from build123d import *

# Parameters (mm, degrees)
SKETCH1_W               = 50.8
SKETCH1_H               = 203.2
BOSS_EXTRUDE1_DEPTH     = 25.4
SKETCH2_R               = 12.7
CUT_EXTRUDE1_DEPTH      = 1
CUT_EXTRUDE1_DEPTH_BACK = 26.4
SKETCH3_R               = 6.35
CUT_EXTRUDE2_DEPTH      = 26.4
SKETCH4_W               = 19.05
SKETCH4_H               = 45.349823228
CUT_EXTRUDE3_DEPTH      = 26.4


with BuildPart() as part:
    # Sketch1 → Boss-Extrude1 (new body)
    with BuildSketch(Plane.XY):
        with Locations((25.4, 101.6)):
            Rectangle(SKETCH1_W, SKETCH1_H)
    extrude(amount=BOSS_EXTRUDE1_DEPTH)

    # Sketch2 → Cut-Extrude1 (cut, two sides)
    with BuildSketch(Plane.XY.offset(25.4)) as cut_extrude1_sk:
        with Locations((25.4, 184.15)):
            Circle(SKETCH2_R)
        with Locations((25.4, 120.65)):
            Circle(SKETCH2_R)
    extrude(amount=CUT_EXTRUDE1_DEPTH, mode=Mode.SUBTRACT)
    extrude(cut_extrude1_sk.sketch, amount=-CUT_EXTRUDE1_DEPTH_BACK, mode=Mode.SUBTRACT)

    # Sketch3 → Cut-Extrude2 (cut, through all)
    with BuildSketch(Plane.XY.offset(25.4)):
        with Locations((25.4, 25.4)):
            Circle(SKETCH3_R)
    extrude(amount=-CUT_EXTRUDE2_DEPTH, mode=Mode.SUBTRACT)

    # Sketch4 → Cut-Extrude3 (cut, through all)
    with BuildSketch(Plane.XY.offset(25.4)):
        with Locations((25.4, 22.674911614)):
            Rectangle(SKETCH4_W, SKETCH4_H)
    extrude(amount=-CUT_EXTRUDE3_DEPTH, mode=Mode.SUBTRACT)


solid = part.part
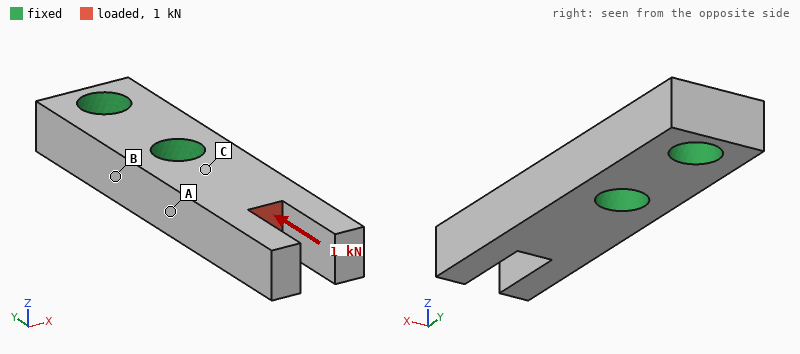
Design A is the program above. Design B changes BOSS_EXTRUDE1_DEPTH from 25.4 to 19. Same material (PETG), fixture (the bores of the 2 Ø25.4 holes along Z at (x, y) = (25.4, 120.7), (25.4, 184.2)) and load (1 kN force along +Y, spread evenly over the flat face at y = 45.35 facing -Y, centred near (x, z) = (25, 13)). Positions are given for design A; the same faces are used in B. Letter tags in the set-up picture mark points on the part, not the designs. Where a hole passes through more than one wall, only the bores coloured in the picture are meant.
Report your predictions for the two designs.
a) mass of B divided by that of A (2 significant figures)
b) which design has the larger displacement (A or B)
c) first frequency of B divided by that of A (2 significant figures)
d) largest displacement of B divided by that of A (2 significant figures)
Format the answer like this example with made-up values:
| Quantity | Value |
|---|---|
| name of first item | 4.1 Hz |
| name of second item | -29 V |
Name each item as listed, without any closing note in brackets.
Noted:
| Quantity | Value |
|---|---|
| mass of B divided by that of A | 0.75 |
| which design has the larger displacement | B |
| first frequency of B divided by that of A | 0.77 |
| largest displacement of B divided by that of A | 1.4 |
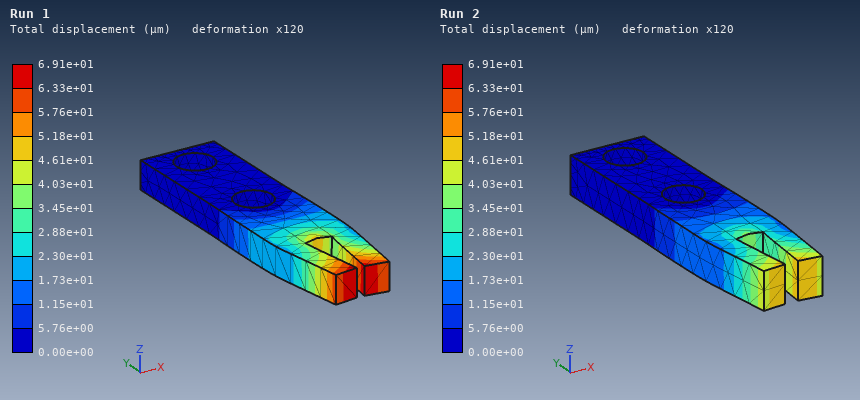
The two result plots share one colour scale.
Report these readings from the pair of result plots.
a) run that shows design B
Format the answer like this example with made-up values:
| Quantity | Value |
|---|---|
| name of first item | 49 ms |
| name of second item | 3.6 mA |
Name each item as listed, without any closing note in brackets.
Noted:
| Quantity | Value |
|---|---|
| run that shows design B | Run 1 |
